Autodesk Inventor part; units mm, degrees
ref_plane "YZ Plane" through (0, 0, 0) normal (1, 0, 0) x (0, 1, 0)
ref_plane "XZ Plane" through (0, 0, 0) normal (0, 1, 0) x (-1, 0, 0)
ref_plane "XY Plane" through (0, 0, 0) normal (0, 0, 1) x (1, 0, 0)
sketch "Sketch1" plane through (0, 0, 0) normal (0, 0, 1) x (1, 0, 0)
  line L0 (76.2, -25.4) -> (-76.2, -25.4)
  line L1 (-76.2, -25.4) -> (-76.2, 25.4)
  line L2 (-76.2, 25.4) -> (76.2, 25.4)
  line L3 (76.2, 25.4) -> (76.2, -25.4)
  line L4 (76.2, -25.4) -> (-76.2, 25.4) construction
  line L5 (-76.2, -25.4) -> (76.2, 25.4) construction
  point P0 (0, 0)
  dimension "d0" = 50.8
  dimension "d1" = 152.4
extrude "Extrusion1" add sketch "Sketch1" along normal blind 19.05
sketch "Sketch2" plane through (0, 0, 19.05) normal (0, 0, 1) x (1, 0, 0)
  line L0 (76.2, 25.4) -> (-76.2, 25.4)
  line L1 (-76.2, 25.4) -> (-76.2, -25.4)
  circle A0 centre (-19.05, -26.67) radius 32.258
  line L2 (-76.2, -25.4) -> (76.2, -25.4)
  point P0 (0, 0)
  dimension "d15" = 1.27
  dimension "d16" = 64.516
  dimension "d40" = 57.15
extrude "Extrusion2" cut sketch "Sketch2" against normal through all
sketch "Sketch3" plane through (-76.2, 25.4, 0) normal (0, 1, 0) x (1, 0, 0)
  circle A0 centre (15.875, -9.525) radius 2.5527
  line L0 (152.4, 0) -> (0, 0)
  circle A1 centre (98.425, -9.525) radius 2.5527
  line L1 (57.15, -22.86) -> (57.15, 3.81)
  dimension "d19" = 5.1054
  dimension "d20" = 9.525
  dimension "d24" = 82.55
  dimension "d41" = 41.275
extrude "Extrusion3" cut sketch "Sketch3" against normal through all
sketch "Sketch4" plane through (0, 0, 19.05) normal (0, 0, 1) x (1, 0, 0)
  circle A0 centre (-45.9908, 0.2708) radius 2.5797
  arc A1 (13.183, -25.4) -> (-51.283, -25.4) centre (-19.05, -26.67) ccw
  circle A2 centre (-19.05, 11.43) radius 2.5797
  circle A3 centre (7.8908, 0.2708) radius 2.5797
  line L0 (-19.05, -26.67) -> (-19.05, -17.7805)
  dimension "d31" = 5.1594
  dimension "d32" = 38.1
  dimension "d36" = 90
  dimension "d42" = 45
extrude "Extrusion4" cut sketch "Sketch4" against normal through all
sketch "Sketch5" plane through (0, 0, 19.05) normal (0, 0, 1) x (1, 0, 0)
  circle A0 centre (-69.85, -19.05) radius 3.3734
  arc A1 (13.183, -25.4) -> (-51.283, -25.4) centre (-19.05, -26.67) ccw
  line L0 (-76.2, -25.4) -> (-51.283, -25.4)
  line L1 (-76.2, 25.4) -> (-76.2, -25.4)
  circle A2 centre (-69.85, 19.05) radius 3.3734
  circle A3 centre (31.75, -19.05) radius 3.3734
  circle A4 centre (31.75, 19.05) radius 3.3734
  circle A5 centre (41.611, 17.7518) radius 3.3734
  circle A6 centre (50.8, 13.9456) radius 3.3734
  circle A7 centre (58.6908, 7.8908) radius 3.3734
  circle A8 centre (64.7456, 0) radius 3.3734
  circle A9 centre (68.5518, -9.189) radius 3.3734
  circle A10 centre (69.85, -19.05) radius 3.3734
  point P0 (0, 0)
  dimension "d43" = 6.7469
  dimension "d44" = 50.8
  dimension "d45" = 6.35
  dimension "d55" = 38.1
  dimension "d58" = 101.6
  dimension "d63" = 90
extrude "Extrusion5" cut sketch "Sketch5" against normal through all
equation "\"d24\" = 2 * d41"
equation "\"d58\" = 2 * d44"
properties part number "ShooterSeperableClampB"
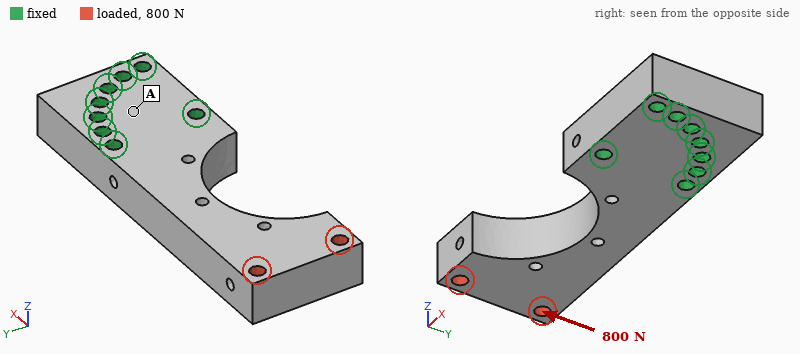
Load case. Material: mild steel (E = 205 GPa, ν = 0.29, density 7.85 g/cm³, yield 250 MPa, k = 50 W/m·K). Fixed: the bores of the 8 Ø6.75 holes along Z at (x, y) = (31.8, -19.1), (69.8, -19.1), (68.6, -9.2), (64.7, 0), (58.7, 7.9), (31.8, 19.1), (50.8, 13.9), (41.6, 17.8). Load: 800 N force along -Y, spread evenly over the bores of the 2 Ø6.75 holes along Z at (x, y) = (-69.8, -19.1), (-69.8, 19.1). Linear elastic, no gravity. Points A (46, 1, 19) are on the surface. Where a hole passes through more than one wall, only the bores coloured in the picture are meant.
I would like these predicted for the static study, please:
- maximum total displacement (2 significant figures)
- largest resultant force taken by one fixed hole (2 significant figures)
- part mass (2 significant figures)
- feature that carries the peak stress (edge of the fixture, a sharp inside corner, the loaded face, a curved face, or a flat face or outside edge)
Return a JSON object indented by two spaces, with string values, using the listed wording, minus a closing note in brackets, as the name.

{
  "maximum total displacement": "62 µm",
  "largest resultant force taken by one fixed hole": "2.1 kN",
  "part mass": "850 g",
  "feature that carries the peak stress": "a curved face"
}
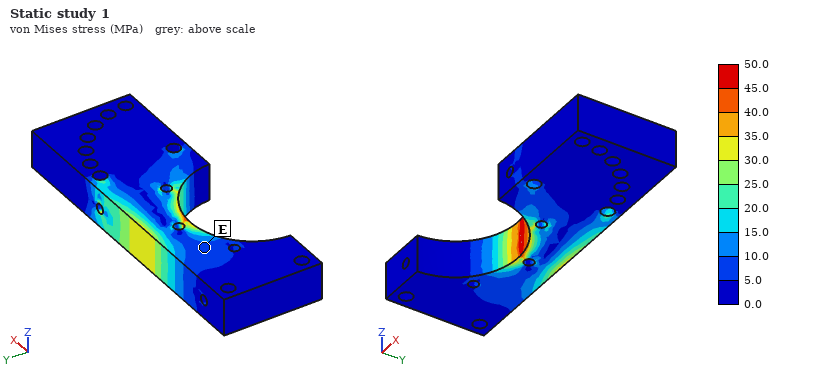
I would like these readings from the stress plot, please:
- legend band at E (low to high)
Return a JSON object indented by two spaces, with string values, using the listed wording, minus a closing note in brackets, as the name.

{
  "legend band at E": "5.0 to 10.0 MPa"
}
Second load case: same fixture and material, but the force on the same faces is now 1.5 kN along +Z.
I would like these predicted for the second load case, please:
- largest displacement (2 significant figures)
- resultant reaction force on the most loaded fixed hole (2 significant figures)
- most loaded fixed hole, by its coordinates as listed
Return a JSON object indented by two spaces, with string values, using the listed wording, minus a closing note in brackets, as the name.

{
  "largest displacement": "0.22 mm",
  "resultant reaction force on the most loaded fixed hole": "1.5 kN",
  "most loaded fixed hole, by its coordinates as listed": "(31.8, 19.1)"
}
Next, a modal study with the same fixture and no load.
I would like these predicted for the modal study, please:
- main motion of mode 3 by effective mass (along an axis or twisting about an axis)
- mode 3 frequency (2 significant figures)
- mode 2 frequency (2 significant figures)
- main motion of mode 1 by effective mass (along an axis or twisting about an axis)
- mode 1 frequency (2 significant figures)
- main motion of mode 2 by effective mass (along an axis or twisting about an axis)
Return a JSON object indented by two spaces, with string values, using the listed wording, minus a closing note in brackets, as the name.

{
  "main motion of mode 3 by effective mass": "twisting about X",
  "mode 3 frequency": "3600 Hz",
  "mode 2 frequency": "1500 Hz",
  "main motion of mode 1 by effective mass": "along Z",
  "mode 1 frequency": "1100 Hz",
  "main motion of mode 2 by effective mass": "along Y"
}
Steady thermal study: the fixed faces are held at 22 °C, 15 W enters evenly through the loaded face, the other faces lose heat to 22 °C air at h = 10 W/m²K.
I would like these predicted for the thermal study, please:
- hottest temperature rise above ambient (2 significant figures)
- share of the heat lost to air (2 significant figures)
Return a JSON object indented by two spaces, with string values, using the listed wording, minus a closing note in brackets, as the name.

{
  "hottest temperature rise above ambient": "53 K",
  "share of the heat lost to air": "28 %"
}
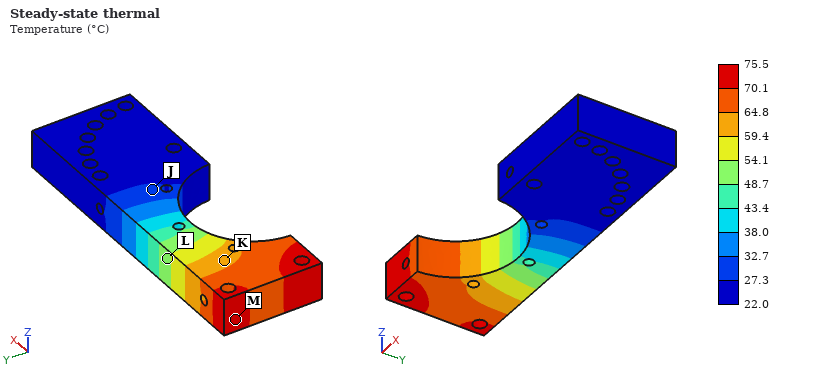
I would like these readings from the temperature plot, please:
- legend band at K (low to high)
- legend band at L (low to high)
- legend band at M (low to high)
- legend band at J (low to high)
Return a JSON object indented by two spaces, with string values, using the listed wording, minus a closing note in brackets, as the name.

{
  "legend band at K": "59.4 to 64.8 °C",
  "legend band at L": "48.7 to 54.1 °C",
  "legend band at M": "70.1 to 75.5 °C",
  "legend band at J": "27.3 to 32.7 °C"
}
